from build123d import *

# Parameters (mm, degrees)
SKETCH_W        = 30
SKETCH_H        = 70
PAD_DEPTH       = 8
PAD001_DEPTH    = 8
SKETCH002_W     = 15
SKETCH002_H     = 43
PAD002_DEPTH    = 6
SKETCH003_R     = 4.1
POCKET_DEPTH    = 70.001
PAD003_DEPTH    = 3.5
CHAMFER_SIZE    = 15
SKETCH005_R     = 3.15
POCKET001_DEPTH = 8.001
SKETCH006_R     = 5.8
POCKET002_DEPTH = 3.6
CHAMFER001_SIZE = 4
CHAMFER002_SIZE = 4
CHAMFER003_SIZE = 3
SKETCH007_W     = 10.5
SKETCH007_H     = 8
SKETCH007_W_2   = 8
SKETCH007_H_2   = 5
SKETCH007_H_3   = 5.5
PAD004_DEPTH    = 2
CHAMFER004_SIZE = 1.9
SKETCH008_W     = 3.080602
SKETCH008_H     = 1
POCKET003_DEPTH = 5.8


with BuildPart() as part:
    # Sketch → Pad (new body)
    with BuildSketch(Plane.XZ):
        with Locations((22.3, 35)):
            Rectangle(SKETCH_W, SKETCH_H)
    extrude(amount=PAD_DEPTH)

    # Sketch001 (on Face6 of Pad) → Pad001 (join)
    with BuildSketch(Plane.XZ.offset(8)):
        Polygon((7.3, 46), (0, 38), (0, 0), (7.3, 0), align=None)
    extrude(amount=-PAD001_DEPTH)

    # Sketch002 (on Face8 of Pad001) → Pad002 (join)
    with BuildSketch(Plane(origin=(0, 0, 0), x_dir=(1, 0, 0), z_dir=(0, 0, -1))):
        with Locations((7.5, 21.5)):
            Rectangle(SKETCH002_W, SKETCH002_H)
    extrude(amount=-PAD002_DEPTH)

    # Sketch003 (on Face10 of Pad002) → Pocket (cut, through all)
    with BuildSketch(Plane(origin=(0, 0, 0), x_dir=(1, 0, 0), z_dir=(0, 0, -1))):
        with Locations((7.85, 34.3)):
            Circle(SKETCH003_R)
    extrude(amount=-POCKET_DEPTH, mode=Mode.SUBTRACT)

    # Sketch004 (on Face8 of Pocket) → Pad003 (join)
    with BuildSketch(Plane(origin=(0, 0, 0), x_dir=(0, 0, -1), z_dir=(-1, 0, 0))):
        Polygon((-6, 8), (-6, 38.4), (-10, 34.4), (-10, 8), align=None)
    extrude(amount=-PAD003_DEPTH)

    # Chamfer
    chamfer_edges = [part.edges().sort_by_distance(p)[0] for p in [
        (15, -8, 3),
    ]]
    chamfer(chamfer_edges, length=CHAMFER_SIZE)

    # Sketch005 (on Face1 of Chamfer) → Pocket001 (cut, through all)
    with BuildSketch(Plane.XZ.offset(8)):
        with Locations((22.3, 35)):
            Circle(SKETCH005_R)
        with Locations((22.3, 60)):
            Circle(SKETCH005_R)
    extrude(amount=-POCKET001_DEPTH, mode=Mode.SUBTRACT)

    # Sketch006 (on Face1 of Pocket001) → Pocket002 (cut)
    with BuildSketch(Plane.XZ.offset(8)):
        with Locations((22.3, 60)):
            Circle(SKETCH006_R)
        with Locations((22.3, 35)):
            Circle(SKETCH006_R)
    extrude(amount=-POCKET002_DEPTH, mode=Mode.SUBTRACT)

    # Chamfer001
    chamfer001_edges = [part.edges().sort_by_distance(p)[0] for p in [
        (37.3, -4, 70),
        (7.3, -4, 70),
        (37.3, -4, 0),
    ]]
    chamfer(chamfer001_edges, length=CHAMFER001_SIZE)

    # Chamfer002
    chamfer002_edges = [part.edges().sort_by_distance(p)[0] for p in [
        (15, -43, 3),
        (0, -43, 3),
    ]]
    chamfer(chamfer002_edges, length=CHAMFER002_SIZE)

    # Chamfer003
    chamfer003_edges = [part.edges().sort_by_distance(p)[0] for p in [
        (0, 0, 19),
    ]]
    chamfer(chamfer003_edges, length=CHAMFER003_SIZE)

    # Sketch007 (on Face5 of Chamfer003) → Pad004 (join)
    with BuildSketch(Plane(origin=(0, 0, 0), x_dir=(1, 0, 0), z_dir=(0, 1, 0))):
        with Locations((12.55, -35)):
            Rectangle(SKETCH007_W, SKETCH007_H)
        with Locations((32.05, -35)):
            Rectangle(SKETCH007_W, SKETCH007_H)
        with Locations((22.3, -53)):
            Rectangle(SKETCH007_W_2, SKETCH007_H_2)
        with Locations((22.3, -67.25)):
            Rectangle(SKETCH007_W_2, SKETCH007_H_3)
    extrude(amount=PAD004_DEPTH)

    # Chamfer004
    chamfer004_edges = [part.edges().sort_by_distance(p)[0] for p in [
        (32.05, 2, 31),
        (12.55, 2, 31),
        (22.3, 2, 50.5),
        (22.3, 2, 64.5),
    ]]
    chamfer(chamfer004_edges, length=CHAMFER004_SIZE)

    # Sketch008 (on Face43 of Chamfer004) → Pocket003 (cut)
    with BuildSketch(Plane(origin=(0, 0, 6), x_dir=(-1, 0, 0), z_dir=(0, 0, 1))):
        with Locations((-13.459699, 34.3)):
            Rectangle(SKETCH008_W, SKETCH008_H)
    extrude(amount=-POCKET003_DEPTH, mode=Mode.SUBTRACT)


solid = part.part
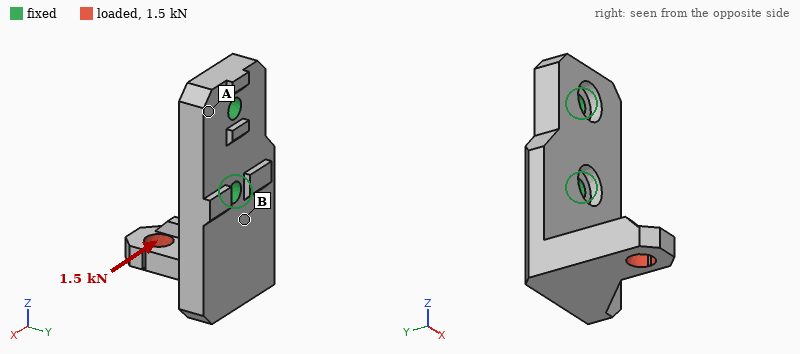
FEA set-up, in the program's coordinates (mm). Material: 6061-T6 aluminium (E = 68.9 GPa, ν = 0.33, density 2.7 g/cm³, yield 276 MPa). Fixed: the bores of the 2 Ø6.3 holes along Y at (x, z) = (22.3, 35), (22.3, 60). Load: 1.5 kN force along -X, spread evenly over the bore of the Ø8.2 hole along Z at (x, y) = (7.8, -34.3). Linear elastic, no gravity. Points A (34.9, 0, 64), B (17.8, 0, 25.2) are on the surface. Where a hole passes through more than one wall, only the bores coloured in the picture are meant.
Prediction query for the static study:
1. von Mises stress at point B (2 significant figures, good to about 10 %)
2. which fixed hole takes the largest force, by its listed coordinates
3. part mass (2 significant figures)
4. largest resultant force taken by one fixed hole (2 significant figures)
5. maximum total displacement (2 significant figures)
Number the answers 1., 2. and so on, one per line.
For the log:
1. 92 MPa
2. (22.3, 35)
3. 60 g
4. 2.7 kN
5. 0.75 mm
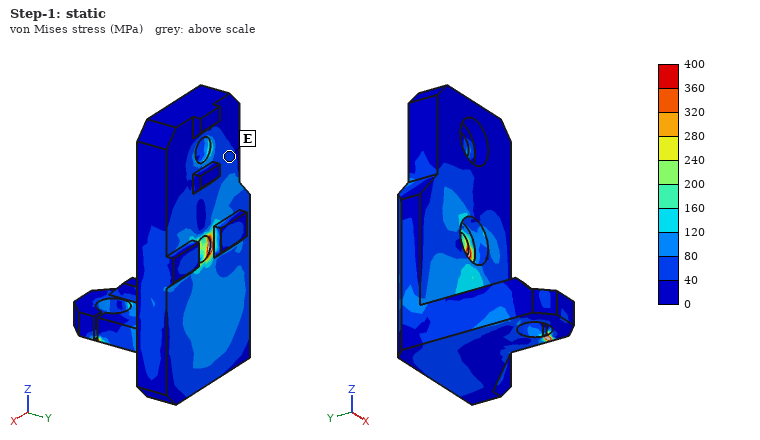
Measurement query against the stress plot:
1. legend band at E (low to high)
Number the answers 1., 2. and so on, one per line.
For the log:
1. 40 to 80 MPa
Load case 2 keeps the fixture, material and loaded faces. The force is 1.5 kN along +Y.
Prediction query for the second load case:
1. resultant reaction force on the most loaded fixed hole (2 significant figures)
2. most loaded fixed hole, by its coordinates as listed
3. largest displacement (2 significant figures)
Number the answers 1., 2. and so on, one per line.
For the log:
1. 3.1 kN
2. (22.3, 35)
3. 0.61 mm
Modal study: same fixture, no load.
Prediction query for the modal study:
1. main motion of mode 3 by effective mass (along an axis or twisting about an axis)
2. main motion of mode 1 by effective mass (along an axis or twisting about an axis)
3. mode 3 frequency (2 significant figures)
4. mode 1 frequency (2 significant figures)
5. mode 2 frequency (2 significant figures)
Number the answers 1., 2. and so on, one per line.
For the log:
1. along Y
2. along Y
3. 5300 Hz
4. 2200 Hz
5. 3400 Hz
